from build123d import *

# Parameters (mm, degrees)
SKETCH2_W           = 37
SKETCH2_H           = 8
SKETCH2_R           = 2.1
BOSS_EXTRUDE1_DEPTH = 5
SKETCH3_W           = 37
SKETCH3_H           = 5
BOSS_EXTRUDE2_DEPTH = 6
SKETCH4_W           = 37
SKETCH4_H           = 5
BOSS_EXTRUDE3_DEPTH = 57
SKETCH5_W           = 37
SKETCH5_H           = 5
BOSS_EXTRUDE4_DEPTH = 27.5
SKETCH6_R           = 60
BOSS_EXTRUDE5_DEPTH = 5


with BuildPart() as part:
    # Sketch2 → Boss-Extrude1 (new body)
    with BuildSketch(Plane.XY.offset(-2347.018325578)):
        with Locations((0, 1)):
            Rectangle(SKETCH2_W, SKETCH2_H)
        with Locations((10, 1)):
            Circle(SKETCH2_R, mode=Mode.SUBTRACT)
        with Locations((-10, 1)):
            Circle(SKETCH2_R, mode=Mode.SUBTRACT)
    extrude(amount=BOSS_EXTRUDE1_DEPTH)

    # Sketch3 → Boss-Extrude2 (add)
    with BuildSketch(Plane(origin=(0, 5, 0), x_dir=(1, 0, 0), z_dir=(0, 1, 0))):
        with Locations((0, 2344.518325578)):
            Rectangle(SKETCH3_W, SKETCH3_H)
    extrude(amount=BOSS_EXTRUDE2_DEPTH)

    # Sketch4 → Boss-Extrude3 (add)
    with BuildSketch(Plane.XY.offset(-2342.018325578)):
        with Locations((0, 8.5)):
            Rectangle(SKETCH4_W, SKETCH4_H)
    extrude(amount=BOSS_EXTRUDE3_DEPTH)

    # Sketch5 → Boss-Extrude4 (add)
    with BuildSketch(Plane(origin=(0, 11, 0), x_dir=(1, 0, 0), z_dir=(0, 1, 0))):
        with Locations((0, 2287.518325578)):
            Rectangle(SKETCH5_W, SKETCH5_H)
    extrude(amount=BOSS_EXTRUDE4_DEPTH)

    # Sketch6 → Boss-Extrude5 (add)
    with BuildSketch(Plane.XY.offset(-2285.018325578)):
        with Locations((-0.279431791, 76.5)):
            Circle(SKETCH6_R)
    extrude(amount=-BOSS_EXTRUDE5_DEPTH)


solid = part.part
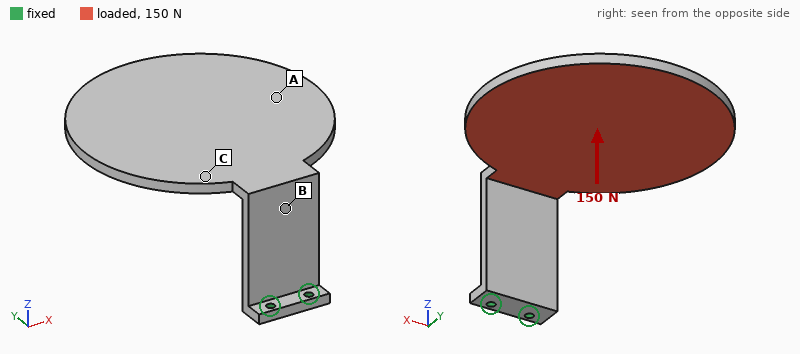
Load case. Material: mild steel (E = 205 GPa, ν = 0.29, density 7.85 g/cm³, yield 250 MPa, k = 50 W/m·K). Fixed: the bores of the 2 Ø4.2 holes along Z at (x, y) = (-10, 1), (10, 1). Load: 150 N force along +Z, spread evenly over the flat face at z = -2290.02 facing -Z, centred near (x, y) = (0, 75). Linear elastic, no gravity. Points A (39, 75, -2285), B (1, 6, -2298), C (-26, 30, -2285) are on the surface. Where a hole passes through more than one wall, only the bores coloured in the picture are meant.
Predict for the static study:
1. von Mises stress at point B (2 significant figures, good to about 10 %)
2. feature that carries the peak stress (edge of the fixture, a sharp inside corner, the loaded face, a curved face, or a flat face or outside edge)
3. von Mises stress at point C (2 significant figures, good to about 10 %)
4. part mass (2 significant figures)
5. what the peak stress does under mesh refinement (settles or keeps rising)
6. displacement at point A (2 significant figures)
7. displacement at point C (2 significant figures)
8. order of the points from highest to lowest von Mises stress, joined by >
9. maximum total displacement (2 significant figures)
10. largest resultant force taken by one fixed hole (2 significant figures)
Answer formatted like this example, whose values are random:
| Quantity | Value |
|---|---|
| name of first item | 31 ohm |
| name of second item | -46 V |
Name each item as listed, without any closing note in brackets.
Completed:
| Quantity | Value |
|---|---|
| von Mises stress at point B | 58 MPa |
| feature that carries the peak stress | edge of the fixture |
| von Mises stress at point C | 20 MPa |
| part mass | 560 g |
| what the peak stress does under mesh refinement | keeps rising |
| displacement at point A | 0.71 mm |
| displacement at point C | 0.33 mm |
| order of the points from highest to lowest von Mises stress, joined by > | B > C > A |
| maximum total displacement | 1.3 mm |
| largest resultant force taken by one fixed hole | 130 N |
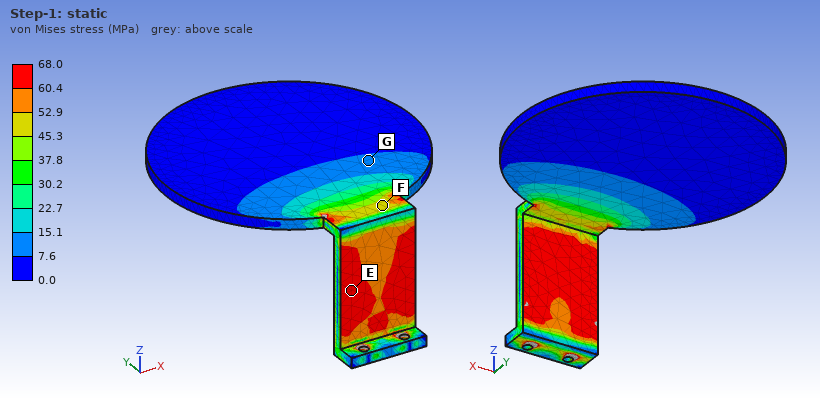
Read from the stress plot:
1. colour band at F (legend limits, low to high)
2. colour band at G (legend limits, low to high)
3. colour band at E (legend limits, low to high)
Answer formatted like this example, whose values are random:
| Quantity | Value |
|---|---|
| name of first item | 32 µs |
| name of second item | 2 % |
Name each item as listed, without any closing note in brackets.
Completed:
| Quantity | Value |
|---|---|
| colour band at F | 45.3 to 52.9 MPa |
| colour band at G | 7.6 to 15.1 MPa |
| colour band at E | 60.4 to 68.0 MPa |
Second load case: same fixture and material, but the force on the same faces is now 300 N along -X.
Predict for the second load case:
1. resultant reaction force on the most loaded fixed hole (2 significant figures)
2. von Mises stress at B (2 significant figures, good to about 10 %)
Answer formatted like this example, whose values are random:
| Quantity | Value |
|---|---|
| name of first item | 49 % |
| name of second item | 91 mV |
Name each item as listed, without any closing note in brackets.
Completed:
| Quantity | Value |
|---|---|
| resultant reaction force on the most loaded fixed hole | 1.2 kN |
| von Mises stress at B | 97 MPa |
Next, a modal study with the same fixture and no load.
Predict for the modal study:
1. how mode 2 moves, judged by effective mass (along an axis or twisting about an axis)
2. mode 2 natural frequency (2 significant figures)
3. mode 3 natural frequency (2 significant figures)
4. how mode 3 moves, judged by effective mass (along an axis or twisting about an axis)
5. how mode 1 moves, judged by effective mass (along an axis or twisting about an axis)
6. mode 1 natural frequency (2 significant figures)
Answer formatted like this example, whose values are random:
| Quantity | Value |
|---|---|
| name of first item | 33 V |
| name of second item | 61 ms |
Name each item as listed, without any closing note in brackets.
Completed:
| Quantity | Value |
|---|---|
| how mode 2 moves, judged by effective mass | along X |
| mode 2 natural frequency | 150 Hz |
| mode 3 natural frequency | 370 Hz |
| how mode 3 moves, judged by effective mass | along Y |
| how mode 1 moves, judged by effective mass | along Z |
| mode 1 natural frequency | 95 Hz |
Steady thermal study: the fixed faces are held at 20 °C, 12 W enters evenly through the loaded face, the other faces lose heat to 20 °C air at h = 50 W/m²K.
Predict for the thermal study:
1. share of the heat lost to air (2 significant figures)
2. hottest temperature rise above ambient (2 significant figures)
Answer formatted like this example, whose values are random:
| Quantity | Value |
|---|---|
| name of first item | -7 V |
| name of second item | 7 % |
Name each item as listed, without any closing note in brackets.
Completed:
| Quantity | Value |
|---|---|
| share of the heat lost to air | 92 % |
| hottest temperature rise above ambient | 16 K |
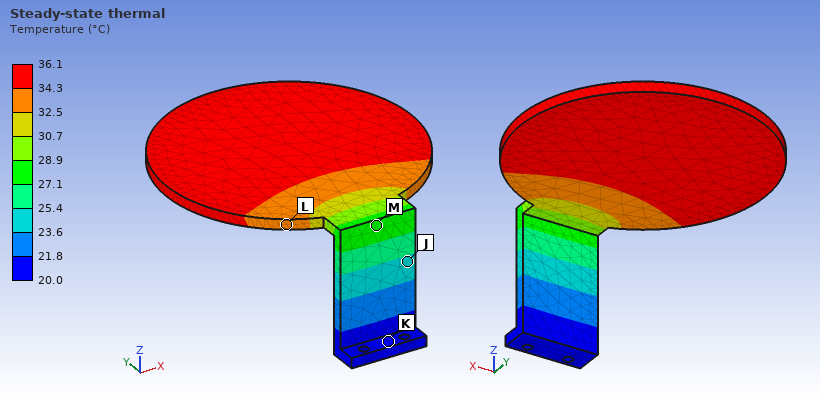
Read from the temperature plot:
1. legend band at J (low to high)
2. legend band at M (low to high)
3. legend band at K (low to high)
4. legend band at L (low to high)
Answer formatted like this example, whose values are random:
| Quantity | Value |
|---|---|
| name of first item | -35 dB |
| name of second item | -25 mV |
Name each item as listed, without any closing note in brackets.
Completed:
| Quantity | Value |
|---|---|
| legend band at J | 23.6 to 25.4 °C |
| legend band at M | 27.1 to 28.9 °C |
| legend band at K | 20.0 to 21.8 °C |
| legend band at L | 32.5 to 34.3 °C |
